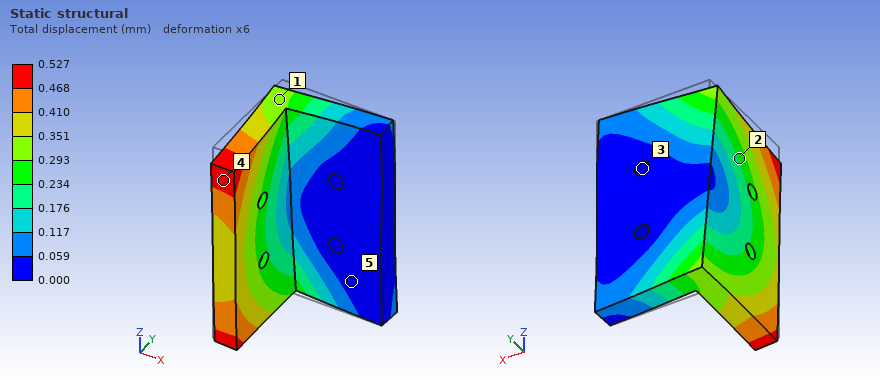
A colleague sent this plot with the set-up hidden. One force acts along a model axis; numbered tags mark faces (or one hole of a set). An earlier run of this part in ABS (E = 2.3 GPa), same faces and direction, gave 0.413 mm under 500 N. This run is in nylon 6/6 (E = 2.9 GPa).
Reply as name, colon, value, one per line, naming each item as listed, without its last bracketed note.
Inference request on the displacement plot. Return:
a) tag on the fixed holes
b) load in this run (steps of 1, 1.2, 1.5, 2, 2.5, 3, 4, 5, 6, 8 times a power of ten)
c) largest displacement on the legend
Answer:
tag on the fixed holes: 3
load in this run: 800 N
largest displacement on the legend: 0.527 mm
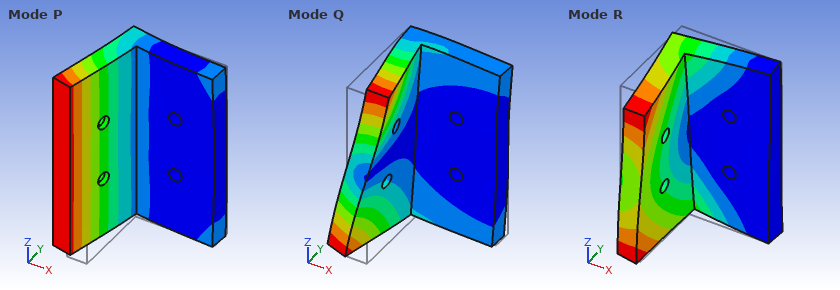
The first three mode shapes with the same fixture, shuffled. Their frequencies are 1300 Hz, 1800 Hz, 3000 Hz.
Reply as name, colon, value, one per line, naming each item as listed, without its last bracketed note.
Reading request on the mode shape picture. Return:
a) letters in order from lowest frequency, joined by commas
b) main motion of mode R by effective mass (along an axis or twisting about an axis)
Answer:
letters in order from lowest frequency, joined by commas: P, R, Q
main motion of mode R by effective mass: along Z
